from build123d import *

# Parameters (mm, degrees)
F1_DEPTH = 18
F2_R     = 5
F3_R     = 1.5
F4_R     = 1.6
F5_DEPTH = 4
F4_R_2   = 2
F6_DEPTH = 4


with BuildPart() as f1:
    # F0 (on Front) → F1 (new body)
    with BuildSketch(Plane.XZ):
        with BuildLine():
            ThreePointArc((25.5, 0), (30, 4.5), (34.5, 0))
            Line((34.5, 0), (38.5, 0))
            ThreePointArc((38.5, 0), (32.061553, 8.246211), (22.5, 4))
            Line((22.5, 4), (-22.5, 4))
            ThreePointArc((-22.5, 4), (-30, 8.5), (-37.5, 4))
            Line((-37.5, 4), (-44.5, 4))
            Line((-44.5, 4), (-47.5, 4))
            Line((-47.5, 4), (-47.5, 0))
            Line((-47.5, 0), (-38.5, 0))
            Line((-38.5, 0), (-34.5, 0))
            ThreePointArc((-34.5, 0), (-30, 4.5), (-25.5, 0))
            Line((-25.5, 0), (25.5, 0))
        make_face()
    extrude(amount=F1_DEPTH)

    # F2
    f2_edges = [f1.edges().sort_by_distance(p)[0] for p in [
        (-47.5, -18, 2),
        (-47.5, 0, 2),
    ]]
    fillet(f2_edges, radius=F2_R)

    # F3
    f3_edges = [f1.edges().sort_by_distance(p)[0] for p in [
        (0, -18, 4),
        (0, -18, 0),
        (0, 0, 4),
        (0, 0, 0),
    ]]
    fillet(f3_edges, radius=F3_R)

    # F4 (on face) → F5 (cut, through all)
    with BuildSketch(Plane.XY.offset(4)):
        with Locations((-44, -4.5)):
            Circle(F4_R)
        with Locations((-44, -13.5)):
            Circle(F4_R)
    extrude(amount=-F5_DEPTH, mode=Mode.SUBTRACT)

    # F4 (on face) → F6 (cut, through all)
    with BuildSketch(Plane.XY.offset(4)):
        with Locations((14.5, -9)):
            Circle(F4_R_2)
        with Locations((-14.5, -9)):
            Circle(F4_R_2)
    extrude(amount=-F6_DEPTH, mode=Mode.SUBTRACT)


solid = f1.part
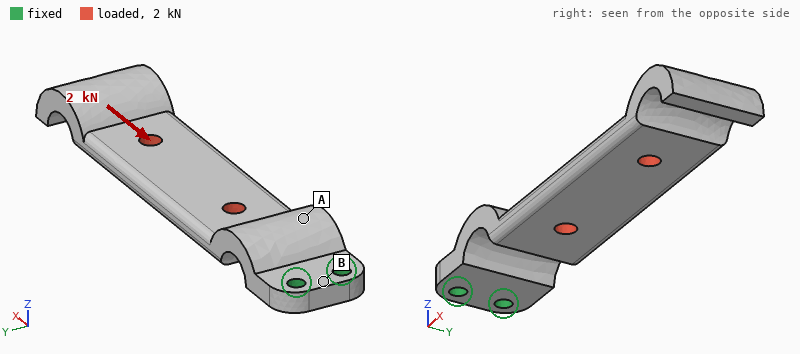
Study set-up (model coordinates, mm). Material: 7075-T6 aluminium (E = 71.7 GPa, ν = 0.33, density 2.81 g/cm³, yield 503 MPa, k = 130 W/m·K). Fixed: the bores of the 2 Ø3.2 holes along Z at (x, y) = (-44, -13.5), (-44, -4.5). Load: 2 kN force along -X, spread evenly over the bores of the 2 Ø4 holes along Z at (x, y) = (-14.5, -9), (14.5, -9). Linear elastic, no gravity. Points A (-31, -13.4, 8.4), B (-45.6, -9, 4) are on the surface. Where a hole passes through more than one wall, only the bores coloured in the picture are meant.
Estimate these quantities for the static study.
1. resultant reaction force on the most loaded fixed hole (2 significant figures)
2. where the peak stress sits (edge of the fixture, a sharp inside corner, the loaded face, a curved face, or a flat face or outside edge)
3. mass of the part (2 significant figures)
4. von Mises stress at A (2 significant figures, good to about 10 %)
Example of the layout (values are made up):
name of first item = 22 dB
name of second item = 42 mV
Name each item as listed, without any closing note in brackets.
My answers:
resultant reaction force on the most loaded fixed hole = 1.0 kN
where the peak stress sits = a curved face
mass of the part = 18 g
von Mises stress at A = 120 MPa
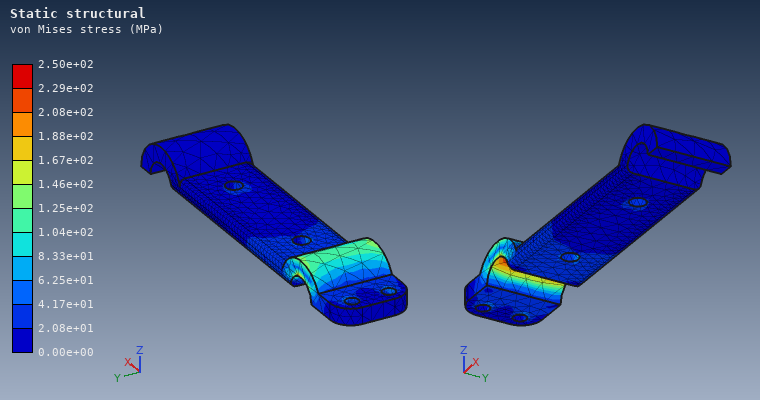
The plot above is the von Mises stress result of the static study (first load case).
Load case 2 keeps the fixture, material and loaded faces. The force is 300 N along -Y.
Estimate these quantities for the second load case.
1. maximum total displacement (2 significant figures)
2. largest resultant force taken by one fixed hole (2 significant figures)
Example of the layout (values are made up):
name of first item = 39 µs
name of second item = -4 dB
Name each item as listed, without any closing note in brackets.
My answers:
maximum total displacement = 0.33 mm
largest resultant force taken by one fixed hole = 1.2 kN
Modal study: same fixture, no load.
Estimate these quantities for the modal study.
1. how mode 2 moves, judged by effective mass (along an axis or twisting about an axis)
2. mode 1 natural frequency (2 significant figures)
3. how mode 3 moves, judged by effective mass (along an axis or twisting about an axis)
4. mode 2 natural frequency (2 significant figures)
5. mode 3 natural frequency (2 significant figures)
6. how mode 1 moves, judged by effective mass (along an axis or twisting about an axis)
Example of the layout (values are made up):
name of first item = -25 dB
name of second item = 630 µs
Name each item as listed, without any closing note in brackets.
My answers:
how mode 2 moves, judged by effective mass = along Y
mode 1 natural frequency = 440 Hz
how mode 3 moves, judged by effective mass = along Z
mode 2 natural frequency = 1400 Hz
mode 3 natural frequency = 2800 Hz
how mode 1 moves, judged by effective mass = along Z
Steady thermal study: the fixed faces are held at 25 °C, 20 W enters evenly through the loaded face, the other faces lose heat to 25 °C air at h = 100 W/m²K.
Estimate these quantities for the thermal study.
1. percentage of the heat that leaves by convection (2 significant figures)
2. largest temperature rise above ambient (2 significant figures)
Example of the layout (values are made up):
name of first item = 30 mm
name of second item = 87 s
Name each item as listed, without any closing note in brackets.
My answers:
percentage of the heat that leaves by convection = 56 %
largest temperature rise above ambient = 44 K
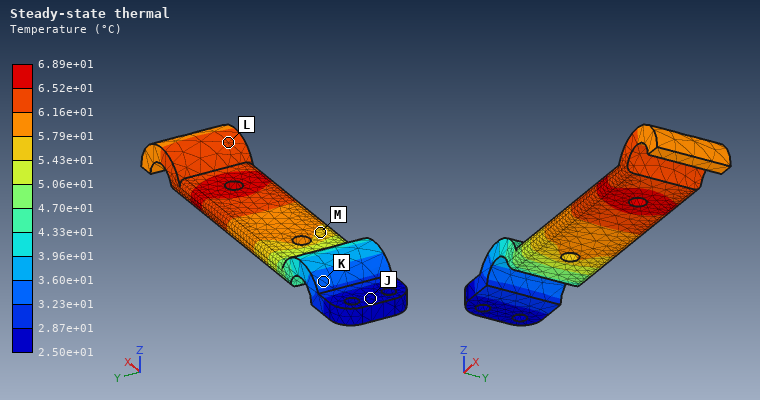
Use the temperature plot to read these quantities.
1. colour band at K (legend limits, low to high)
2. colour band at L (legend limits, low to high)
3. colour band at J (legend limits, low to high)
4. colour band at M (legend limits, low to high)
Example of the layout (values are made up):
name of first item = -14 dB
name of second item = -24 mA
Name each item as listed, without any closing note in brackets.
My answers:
colour band at K = 3.23e+01 to 3.60e+01 °C
colour band at L = 6.16e+01 to 6.52e+01 °C
colour band at J = 2.50e+01 to 2.87e+01 °C
colour band at M = 5.43e+01 to 5.79e+01 °C
